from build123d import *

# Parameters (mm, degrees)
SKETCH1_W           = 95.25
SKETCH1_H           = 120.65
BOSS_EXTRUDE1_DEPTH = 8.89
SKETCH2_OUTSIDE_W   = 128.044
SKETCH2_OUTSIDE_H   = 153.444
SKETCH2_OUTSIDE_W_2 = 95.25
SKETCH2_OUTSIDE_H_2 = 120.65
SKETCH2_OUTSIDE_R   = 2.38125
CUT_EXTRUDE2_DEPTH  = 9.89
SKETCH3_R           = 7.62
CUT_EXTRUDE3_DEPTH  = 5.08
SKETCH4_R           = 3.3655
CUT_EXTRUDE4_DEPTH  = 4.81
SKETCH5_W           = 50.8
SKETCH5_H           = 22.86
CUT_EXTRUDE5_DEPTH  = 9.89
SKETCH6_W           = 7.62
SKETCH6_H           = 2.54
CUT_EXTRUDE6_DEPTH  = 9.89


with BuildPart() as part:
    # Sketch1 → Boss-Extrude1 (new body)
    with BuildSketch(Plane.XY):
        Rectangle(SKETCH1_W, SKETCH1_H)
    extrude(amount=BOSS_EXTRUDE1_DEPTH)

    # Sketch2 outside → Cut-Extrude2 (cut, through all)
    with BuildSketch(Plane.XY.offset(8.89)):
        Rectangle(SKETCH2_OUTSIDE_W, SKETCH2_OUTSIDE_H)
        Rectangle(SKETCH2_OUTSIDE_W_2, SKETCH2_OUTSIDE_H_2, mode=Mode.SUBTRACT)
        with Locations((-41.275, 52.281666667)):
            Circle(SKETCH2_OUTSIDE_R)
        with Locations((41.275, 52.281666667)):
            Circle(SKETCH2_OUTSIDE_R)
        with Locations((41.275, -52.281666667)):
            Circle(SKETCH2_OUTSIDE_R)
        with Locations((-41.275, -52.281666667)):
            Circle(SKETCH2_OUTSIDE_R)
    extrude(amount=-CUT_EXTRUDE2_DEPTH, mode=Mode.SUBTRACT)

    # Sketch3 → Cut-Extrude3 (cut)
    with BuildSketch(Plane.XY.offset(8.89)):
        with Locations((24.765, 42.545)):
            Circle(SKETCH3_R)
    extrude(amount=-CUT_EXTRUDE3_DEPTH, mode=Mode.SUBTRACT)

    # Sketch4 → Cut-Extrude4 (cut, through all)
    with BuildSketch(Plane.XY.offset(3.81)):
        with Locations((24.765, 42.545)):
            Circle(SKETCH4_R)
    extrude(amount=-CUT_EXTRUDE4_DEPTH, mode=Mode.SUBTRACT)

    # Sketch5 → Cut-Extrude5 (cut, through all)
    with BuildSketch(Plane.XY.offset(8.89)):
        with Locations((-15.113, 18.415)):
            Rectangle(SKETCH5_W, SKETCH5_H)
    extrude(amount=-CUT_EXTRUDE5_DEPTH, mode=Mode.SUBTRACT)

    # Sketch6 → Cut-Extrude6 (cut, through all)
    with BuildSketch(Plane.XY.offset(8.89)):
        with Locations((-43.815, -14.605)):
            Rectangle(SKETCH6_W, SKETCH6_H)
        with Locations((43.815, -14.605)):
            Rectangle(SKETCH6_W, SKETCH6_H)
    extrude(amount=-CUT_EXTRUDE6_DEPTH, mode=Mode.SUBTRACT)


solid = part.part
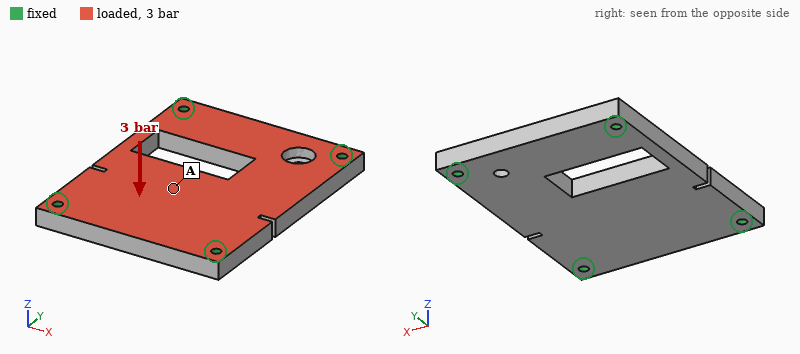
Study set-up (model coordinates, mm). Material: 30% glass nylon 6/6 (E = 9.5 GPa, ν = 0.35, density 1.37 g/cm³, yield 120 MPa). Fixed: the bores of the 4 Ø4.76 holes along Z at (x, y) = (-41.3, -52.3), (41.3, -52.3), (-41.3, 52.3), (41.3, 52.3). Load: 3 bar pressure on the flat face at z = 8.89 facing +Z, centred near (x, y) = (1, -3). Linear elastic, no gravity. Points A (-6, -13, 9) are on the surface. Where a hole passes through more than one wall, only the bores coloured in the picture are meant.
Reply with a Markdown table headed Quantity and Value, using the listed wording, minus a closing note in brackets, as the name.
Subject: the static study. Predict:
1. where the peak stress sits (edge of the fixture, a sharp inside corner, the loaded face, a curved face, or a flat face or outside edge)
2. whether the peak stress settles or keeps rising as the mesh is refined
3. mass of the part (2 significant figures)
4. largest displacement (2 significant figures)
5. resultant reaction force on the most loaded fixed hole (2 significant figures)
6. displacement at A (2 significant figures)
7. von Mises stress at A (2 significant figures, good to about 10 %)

| Quantity | Value |
|---|---|
| where the peak stress sits | edge of the fixture |
| whether the peak stress settles or keeps rising as the mesh is refined | keeps rising |
| mass of the part | 120 g |
| largest displacement | 0.50 mm |
| resultant reaction force on the most loaded fixed hole | 810 N |
| displacement at A | 0.39 mm |
| von Mises stress at A | 9.2 MPa |
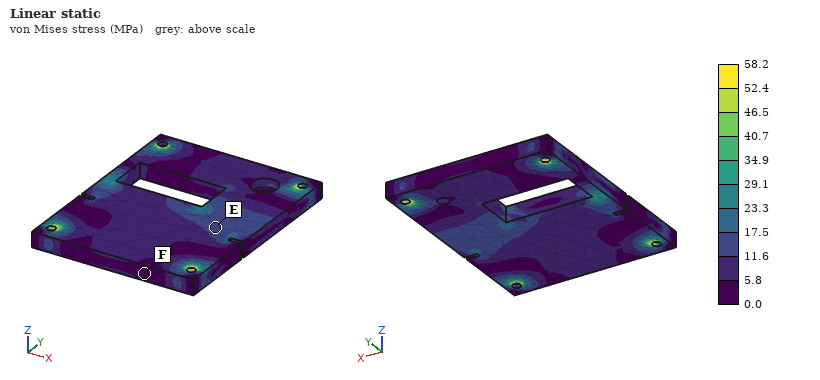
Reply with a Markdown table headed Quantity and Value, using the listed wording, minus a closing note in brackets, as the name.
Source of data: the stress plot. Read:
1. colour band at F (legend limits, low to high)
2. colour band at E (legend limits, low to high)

| Quantity | Value |
|---|---|
| colour band at F | 0.0 to 5.8 MPa |
| colour band at E | 11.6 to 17.5 MPa |
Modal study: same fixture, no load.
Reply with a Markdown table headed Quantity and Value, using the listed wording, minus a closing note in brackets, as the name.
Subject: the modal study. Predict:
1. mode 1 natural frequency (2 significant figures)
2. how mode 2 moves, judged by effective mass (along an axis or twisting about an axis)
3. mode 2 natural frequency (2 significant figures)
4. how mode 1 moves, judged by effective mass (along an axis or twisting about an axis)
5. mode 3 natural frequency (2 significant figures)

| Quantity | Value |
|---|---|
| mode 1 natural frequency | 1400 Hz |
| how mode 2 moves, judged by effective mass | twisting about Y |
| mode 2 natural frequency | 2300 Hz |
| how mode 1 moves, judged by effective mass | along Z |
| mode 3 natural frequency | 3000 Hz |
